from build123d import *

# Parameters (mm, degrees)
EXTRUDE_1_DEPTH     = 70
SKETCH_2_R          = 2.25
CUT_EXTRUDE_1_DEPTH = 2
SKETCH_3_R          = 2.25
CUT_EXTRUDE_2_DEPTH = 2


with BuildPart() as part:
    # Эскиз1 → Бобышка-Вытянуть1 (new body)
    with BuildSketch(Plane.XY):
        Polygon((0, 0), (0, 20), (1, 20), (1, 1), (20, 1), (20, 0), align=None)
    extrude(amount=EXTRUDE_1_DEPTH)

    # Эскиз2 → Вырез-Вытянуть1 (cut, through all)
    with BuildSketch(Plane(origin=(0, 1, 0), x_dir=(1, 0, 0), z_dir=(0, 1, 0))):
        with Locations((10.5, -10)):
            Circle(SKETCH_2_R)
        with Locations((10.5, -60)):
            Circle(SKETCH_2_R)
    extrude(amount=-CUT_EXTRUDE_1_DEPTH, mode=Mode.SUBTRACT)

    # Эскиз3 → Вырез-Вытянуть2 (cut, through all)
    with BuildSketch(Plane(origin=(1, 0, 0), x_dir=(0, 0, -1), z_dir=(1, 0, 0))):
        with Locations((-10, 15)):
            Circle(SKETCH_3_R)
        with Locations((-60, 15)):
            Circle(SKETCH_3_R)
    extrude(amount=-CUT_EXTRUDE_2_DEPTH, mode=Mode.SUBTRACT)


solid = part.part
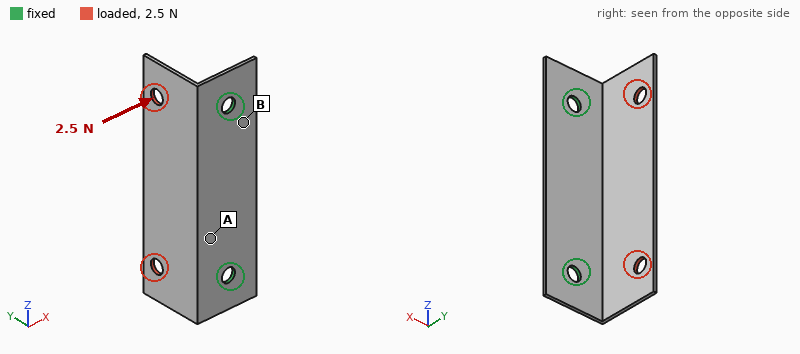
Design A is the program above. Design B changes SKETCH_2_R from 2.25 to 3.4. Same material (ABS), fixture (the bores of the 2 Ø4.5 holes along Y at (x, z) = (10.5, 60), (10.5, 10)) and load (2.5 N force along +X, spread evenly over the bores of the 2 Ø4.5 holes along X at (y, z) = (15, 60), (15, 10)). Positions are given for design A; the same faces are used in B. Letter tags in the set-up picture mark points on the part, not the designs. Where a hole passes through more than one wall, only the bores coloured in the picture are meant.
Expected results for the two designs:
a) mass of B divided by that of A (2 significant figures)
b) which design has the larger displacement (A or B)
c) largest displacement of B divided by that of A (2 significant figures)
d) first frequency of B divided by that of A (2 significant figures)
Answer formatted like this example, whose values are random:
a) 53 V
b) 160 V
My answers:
a) 0.98
b) A
c) 0.88
d) 1.1
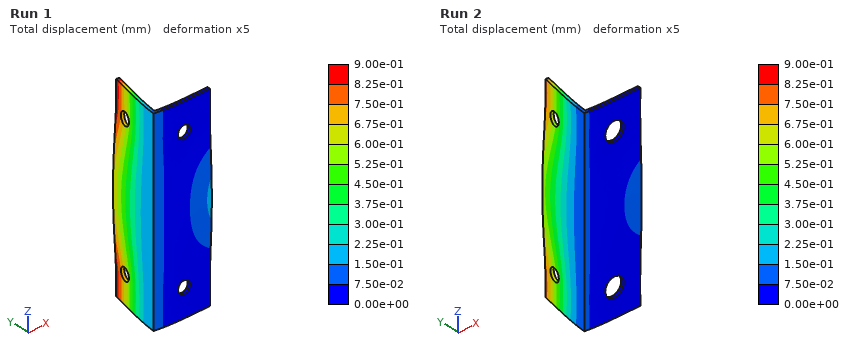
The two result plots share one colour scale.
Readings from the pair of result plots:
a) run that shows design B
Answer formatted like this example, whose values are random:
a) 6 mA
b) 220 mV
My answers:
a) Run 2
